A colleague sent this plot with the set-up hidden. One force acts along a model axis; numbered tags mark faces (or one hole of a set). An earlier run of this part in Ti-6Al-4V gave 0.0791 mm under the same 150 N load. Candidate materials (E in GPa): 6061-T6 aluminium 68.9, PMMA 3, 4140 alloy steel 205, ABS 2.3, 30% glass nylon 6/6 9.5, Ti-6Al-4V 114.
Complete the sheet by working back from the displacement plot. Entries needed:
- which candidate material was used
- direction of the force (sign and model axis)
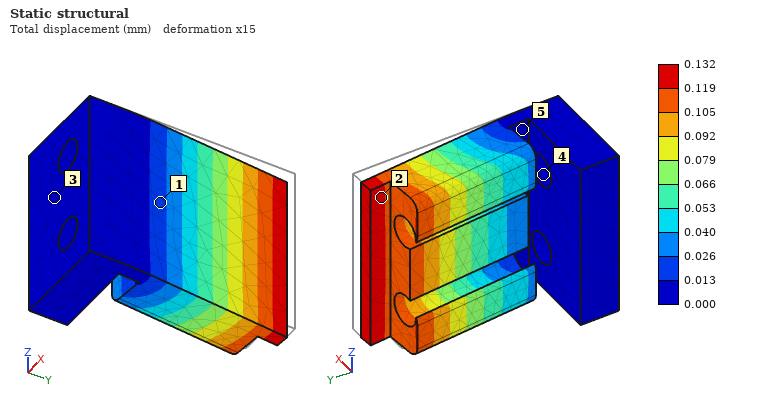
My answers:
6061-T6 aluminium
-X
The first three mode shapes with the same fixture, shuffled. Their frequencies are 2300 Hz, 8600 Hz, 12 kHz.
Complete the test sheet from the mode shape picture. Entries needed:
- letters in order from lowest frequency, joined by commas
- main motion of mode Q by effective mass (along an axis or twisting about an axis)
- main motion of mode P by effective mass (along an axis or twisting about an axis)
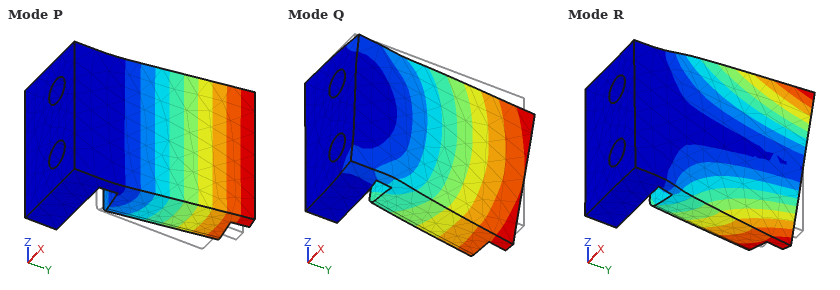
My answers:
P, R, Q
along Z
along X
